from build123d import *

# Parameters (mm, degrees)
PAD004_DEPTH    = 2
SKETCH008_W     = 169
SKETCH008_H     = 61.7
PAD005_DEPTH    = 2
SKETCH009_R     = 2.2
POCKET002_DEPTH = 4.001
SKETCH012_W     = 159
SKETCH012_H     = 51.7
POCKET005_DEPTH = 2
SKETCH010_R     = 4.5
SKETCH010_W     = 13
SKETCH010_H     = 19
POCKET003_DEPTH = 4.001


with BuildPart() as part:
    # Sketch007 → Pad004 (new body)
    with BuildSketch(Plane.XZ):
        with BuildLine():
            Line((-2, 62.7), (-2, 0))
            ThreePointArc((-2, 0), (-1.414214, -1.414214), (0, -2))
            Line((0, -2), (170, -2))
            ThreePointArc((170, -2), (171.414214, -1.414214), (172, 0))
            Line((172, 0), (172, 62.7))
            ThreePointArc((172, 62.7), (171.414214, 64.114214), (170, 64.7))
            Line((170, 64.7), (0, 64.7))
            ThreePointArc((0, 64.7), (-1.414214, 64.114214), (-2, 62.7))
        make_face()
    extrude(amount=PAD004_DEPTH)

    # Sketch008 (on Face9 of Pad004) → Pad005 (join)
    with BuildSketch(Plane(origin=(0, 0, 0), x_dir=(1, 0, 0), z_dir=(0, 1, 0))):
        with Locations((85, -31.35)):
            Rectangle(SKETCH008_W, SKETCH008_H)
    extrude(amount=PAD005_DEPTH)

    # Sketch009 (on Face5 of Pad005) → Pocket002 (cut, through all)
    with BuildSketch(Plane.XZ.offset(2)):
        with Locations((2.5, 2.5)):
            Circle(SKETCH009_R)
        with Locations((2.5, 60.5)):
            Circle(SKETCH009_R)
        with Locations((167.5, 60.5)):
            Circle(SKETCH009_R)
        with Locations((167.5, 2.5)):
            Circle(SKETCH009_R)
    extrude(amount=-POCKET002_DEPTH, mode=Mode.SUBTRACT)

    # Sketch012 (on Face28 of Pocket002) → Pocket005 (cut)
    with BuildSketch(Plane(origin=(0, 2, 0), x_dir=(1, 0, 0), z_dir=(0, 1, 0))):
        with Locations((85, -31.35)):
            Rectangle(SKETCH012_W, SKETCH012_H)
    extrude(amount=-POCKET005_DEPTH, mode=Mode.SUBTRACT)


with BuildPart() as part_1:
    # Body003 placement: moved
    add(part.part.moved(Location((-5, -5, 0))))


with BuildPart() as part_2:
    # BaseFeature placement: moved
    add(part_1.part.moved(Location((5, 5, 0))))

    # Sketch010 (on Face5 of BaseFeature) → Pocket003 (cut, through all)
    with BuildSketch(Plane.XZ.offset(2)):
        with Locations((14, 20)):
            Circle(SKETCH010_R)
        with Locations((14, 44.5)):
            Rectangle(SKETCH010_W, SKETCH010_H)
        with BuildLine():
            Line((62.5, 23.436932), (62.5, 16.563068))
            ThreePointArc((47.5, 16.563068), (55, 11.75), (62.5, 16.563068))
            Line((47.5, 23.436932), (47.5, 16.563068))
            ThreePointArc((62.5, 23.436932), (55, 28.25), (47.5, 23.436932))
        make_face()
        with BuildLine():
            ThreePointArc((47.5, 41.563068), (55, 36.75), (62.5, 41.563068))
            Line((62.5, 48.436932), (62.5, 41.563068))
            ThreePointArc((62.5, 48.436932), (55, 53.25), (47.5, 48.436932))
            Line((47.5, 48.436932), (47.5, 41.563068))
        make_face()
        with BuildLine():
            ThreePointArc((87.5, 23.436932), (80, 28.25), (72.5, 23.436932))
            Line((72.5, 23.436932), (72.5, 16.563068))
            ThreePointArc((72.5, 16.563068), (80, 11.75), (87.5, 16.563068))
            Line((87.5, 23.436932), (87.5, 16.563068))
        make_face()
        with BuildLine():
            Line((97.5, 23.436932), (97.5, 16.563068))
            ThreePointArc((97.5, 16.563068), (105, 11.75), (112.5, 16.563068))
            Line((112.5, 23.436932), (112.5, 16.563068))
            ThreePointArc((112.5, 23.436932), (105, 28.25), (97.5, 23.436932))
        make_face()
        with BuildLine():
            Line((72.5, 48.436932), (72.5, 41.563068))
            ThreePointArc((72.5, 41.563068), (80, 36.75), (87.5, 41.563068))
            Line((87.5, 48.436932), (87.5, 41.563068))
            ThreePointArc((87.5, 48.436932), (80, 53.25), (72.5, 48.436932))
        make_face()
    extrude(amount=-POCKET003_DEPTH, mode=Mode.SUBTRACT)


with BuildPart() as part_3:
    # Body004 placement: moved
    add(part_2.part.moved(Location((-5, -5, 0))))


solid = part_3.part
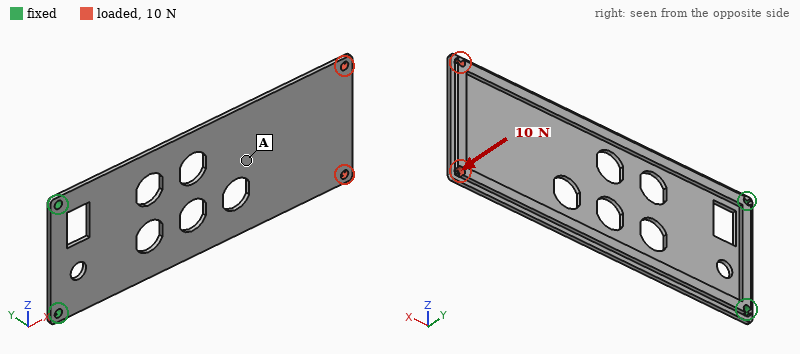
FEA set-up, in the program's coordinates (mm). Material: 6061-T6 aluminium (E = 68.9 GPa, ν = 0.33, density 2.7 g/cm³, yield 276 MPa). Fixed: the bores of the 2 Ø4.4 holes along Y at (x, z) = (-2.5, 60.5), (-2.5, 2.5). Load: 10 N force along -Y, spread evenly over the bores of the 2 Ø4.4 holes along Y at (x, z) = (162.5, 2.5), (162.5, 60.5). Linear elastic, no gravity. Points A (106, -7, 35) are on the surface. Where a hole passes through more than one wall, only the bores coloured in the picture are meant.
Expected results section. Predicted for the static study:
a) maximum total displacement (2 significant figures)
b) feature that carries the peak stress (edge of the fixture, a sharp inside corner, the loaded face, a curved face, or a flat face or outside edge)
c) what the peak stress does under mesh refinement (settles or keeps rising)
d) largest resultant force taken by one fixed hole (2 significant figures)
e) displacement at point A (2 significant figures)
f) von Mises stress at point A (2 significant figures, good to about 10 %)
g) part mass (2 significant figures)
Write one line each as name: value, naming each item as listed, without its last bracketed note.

maximum total displacement: 2.2 mm
feature that carries the peak stress: edge of the fixture
what the peak stress does under mesh refinement: keeps rising
largest resultant force taken by one fixed hole: 31 N
displacement at point A: 1.1 mm
von Mises stress at point A: 6.7 MPa
part mass: 67 g
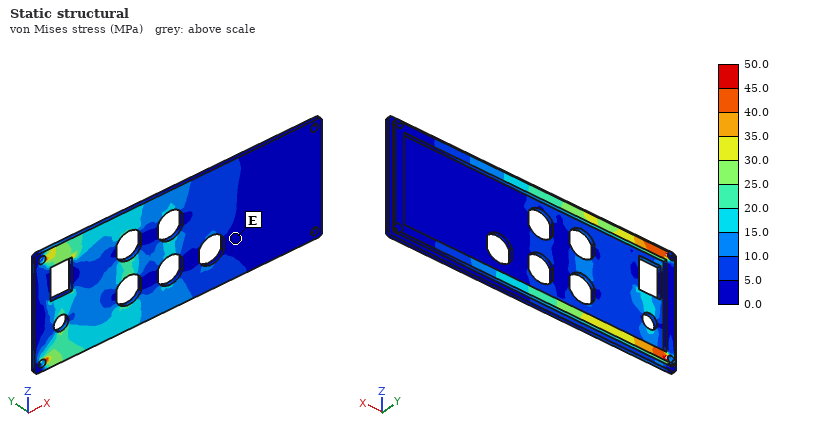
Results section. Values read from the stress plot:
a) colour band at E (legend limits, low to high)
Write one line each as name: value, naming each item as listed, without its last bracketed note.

colour band at E: 0.0 to 5.0 MPa
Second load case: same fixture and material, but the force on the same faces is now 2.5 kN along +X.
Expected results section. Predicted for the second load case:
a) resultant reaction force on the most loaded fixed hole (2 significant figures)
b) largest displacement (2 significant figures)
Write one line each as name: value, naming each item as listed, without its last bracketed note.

resultant reaction force on the most loaded fixed hole: 1.3 kN
largest displacement: 1.9 mm
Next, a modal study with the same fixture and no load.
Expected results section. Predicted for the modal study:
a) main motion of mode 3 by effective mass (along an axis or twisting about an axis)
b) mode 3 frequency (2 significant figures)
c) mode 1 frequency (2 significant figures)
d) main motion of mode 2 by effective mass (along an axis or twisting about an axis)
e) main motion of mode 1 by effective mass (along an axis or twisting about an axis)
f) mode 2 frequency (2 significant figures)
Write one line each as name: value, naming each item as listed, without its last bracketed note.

main motion of mode 3 by effective mass: along Y
mode 3 frequency: 530 Hz
mode 1 frequency: 79 Hz
main motion of mode 2 by effective mass: twisting about X
main motion of mode 1 by effective mass: along Y
mode 2 frequency: 350 Hz
